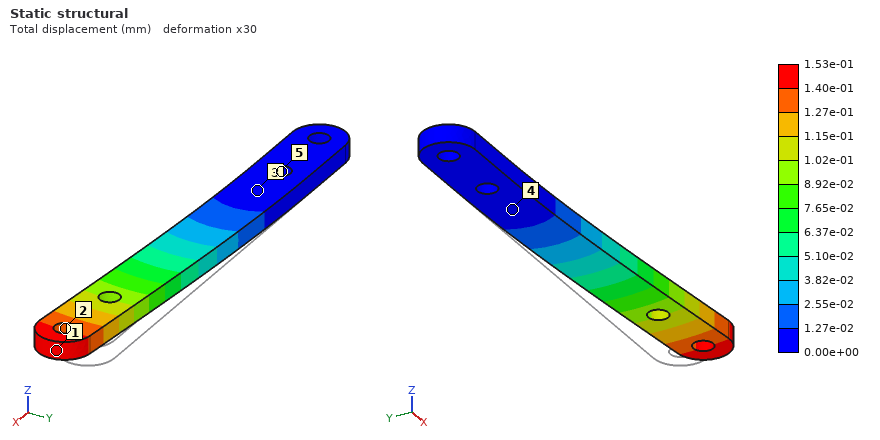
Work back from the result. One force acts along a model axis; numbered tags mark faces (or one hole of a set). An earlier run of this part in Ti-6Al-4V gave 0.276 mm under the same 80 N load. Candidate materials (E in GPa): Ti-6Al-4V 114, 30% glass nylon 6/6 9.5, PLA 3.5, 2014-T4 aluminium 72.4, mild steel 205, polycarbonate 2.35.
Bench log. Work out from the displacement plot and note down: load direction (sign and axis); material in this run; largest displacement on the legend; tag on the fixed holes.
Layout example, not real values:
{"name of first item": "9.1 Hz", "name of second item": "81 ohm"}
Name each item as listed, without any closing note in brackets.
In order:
{"load direction": "-Y", "material in this run": "mild steel", "largest displacement on the legend": "1.53e-01 mm", "tag on the fixed holes": "5"}
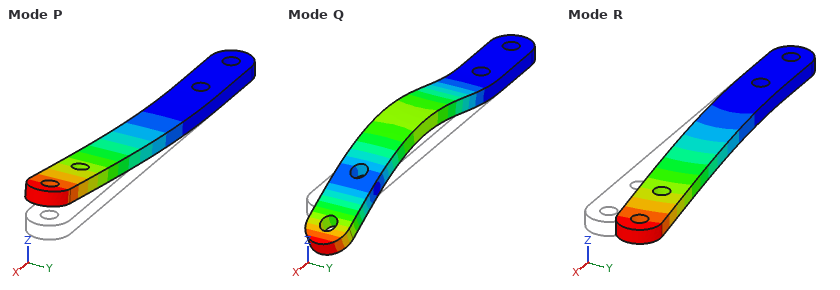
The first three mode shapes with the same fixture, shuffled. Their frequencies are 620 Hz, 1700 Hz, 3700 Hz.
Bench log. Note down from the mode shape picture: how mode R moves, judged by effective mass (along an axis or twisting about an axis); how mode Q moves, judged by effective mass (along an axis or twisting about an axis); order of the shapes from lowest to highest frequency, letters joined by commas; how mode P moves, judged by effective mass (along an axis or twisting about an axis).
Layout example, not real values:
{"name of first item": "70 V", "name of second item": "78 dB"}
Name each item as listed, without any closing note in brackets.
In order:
{"how mode R moves, judged by effective mass": "along Y", "how mode Q moves, judged by effective mass": "along Z", "order of the shapes from lowest to highest frequency, letters joined by commas": "P, R, Q", "how mode P moves, judged by effective mass": "along Z"}
